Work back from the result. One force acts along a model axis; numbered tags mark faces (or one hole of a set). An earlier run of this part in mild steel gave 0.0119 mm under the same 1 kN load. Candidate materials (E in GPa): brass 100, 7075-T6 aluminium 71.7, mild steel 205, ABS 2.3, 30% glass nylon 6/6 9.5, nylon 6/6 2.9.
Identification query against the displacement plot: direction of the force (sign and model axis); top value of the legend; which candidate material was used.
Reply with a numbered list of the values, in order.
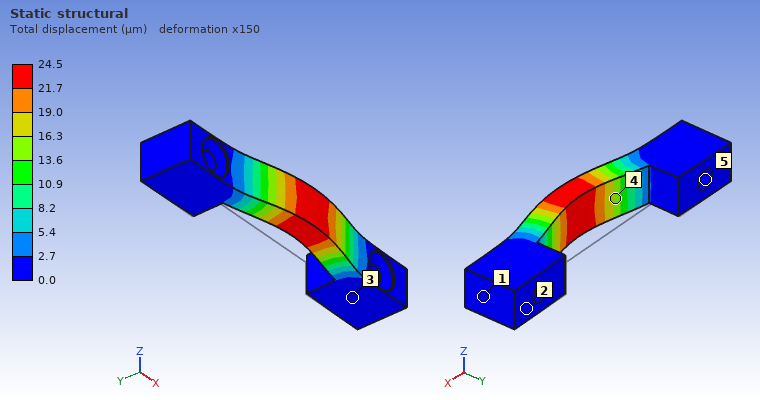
1. -Y
2. 24.5 µm
3. brass
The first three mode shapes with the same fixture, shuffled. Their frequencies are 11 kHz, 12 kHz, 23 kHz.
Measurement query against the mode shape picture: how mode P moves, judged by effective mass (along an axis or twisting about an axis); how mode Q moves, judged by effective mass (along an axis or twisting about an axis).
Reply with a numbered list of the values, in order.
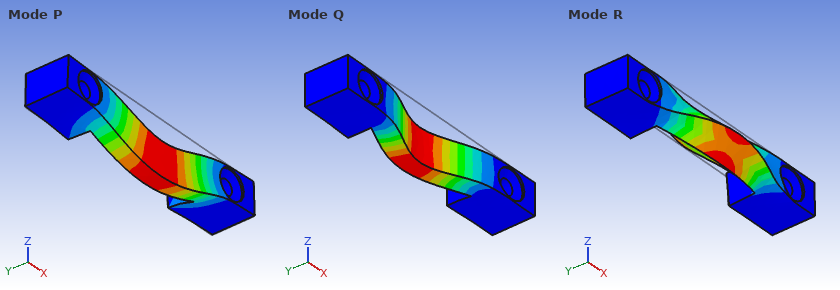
1. along Z
2. along Y
